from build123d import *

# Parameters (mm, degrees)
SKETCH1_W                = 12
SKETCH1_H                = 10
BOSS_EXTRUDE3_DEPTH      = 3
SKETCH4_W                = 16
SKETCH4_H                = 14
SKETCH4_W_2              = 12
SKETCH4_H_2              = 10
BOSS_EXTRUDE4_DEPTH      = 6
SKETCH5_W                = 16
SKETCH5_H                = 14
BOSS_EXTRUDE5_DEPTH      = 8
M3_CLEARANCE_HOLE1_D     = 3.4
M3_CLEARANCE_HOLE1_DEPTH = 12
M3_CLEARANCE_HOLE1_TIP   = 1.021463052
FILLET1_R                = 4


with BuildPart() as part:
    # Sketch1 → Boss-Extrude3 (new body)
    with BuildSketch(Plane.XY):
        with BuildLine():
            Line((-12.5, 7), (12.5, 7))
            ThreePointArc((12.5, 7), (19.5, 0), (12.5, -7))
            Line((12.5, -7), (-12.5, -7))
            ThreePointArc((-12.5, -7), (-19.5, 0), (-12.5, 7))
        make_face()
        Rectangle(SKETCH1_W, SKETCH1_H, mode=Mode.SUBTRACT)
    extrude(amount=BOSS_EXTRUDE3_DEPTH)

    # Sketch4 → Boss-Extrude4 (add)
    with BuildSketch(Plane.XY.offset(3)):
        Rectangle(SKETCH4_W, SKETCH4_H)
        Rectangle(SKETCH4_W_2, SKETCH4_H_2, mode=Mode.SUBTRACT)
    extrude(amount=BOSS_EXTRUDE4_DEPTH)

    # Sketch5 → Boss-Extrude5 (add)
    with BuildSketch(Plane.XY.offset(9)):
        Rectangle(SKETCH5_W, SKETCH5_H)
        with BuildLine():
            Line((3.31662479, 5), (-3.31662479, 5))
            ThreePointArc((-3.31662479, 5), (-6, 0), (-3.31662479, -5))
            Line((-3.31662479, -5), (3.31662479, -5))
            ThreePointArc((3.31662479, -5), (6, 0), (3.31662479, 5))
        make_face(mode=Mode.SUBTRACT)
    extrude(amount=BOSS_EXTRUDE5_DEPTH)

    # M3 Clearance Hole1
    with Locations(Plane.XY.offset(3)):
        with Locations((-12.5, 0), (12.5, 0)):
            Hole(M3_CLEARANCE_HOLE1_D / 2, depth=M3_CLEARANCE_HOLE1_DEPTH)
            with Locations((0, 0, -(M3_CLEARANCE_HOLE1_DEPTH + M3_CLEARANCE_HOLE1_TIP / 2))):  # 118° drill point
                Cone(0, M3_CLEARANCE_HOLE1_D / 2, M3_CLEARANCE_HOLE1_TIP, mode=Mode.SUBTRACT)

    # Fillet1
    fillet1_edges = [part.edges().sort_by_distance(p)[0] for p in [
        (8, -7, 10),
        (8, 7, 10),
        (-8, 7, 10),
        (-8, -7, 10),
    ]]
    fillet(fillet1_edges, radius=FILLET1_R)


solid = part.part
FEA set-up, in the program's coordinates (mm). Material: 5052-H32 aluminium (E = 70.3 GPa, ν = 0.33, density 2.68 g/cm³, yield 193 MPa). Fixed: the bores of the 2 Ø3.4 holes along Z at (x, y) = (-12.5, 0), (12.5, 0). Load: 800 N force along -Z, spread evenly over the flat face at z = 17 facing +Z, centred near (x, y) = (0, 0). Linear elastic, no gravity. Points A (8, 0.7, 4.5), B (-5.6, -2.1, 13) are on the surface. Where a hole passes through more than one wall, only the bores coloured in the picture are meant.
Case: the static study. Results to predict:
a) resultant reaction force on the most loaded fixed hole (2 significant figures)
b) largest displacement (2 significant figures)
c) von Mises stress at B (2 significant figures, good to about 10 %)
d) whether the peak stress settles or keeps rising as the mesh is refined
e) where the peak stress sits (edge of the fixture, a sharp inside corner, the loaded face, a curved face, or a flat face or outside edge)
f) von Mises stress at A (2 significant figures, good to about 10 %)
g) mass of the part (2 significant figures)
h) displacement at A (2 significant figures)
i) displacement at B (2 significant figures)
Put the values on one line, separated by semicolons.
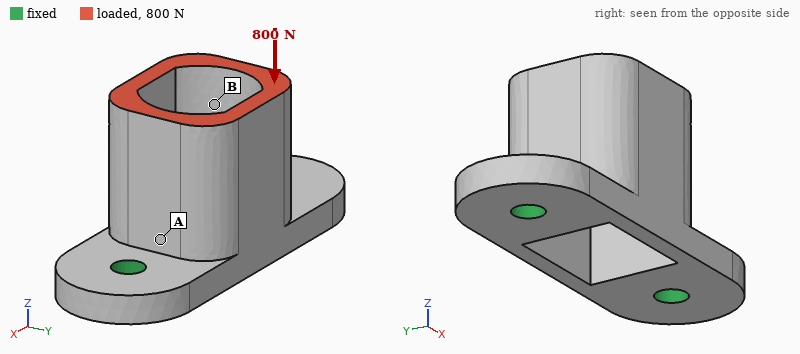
420 N; 9.8 µm; 13 MPa; keeps rising; edge of the fixture; 43 MPa; 6.7 g; 7.2 µm; 8.9 µm
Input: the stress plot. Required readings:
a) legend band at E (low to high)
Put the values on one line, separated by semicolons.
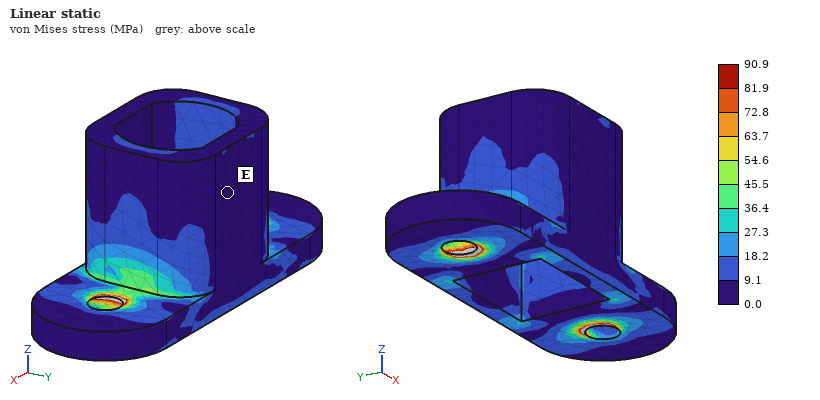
0.0 to 9.1 MPa
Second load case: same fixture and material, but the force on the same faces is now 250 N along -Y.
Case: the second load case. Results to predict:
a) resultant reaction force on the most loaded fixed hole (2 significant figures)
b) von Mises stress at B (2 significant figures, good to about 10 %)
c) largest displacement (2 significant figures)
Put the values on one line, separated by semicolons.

130 N; 13 MPa; 55 µm
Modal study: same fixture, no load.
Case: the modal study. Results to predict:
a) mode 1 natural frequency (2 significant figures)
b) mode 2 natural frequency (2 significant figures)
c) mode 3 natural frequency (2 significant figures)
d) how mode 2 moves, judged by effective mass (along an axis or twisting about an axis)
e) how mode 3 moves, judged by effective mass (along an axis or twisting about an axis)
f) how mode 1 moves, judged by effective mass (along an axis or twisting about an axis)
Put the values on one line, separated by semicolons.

8300 Hz; 19 kHz; 22 kHz; along X; along Z; along Y
